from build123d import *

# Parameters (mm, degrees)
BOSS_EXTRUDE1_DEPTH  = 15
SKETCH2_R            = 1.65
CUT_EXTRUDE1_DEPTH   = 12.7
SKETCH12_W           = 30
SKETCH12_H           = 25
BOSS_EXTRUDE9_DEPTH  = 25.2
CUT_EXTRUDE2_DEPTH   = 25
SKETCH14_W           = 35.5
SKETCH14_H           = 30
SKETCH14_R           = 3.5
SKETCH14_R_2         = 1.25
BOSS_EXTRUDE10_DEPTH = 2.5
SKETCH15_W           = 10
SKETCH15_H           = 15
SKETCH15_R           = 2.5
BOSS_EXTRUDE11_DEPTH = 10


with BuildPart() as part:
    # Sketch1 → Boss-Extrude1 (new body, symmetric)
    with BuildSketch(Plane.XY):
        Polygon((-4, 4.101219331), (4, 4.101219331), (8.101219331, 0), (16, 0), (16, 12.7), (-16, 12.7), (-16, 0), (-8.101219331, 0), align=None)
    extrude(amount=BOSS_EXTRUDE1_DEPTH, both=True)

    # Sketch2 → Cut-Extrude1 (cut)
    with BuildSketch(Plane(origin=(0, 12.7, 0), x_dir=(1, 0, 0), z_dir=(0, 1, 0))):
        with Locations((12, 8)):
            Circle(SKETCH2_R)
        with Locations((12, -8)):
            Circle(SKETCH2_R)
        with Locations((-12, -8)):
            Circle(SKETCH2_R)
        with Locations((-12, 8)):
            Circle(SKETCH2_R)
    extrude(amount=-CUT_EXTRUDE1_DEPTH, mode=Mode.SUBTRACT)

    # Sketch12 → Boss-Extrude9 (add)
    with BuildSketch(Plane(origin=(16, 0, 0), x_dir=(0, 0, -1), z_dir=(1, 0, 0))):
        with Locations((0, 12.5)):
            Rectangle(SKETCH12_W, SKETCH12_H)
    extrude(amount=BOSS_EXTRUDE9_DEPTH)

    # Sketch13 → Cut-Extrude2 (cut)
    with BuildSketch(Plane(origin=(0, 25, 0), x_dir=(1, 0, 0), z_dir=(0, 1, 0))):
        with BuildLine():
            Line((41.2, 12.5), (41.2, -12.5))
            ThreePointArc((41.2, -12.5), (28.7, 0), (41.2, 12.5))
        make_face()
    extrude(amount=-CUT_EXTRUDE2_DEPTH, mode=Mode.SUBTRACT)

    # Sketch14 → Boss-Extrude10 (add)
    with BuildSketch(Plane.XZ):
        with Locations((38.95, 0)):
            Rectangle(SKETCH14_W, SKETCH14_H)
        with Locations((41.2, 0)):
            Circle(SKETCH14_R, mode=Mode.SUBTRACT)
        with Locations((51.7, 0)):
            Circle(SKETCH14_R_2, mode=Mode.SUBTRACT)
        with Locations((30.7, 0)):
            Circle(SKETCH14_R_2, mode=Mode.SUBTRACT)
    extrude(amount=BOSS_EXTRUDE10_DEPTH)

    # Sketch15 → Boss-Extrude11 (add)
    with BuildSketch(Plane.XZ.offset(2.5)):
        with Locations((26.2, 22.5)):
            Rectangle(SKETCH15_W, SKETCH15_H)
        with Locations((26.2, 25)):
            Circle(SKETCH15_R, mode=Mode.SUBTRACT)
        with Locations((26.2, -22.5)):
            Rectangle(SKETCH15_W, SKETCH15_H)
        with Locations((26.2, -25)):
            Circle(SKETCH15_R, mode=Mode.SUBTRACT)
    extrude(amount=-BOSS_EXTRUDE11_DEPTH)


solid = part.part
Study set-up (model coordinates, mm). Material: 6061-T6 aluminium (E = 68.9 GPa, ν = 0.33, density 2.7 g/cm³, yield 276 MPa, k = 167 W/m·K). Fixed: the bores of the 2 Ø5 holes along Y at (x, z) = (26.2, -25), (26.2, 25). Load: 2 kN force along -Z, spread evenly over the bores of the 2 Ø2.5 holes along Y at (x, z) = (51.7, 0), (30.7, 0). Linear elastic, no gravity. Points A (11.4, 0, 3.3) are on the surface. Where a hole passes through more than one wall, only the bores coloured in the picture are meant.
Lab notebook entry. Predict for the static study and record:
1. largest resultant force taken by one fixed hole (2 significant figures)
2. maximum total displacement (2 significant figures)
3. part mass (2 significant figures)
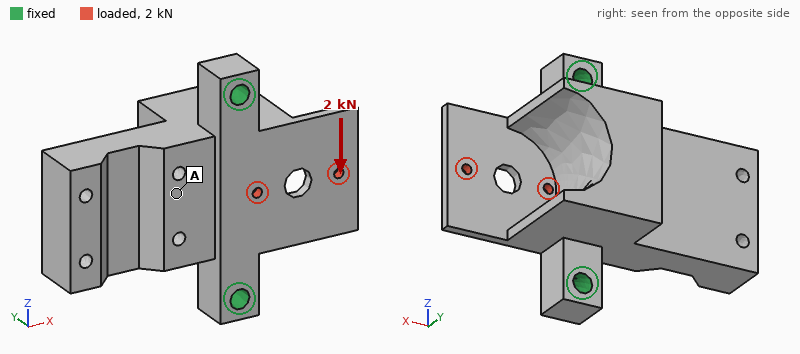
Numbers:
1.2 kN
40 µm
76 g
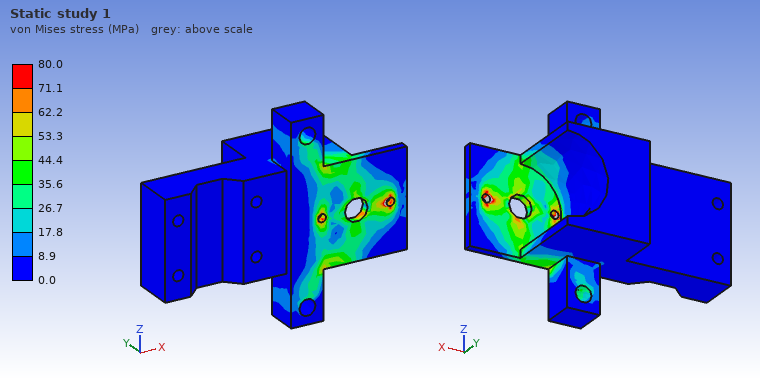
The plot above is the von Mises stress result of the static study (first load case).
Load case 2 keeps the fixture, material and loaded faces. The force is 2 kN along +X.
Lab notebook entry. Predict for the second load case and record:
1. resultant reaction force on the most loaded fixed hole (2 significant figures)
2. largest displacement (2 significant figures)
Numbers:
1.0 kN
52 µm
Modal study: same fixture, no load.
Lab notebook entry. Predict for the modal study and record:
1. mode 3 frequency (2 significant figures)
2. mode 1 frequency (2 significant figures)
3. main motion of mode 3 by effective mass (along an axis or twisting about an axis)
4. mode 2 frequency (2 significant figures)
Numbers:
7400 Hz
2300 Hz
along Z
4800 Hz
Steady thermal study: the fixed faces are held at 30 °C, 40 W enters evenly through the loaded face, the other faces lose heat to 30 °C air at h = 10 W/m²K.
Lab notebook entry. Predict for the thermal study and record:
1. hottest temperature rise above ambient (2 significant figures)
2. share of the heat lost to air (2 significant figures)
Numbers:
64 K
3.9 %
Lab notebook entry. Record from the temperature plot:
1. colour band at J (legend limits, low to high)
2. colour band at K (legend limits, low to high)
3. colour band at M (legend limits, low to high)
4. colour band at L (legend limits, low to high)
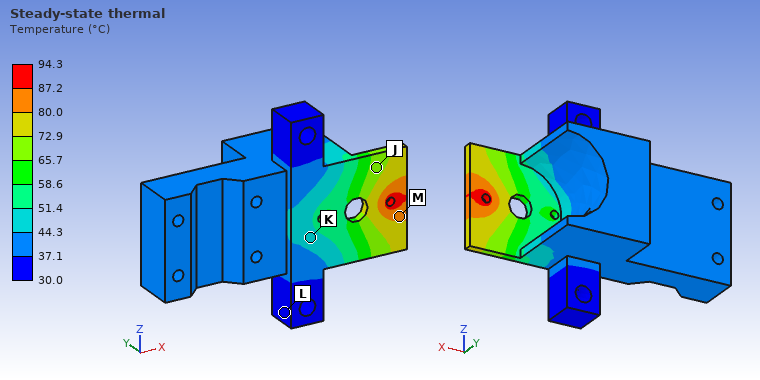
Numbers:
65.7 to 72.9 °C
44.3 to 51.4 °C
80.0 to 87.2 °C
30.0 to 37.1 °C
